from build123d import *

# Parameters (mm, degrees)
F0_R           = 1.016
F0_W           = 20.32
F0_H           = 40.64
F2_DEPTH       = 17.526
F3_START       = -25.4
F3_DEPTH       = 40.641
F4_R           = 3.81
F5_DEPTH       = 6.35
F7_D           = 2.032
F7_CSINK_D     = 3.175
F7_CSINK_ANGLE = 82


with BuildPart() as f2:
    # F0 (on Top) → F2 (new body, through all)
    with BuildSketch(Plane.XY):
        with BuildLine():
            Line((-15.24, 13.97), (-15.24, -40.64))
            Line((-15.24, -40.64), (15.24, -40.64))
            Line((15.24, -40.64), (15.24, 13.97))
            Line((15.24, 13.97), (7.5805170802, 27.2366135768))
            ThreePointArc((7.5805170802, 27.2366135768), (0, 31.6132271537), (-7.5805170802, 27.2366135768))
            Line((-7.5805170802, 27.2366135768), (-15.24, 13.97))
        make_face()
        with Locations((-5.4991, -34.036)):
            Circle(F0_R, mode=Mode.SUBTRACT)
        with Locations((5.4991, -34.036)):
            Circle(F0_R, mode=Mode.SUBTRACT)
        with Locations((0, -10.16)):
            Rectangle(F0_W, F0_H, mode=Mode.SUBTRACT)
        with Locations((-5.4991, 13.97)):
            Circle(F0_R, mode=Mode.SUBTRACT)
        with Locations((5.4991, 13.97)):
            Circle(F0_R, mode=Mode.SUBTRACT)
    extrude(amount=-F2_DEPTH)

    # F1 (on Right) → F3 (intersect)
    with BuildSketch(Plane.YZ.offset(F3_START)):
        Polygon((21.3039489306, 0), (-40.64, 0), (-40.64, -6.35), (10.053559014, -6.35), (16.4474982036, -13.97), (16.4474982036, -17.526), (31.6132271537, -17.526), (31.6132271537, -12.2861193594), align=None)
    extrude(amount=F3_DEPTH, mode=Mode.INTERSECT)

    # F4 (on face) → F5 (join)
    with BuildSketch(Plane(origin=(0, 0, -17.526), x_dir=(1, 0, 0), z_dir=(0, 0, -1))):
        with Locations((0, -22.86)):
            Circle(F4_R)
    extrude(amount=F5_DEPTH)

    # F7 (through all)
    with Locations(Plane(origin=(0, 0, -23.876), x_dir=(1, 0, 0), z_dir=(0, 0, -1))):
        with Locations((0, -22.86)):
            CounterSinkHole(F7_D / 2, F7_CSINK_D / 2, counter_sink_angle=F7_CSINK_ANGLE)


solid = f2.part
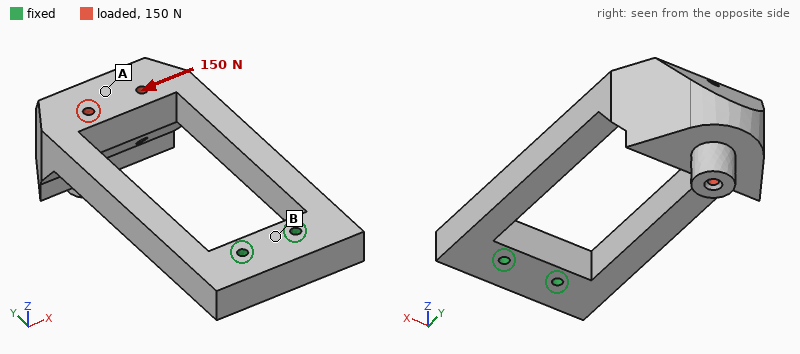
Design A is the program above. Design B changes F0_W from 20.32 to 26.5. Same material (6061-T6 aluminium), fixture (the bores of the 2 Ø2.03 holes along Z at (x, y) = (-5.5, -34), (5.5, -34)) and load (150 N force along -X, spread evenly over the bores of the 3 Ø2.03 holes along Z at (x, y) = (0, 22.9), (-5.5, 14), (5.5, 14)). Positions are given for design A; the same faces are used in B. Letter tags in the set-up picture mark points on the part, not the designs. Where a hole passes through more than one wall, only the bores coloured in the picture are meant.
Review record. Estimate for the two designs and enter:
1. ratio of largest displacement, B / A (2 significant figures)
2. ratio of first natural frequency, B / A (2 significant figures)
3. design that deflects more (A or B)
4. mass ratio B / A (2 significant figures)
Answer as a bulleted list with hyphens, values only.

- 8.3
- 0.60
- B
- 0.85
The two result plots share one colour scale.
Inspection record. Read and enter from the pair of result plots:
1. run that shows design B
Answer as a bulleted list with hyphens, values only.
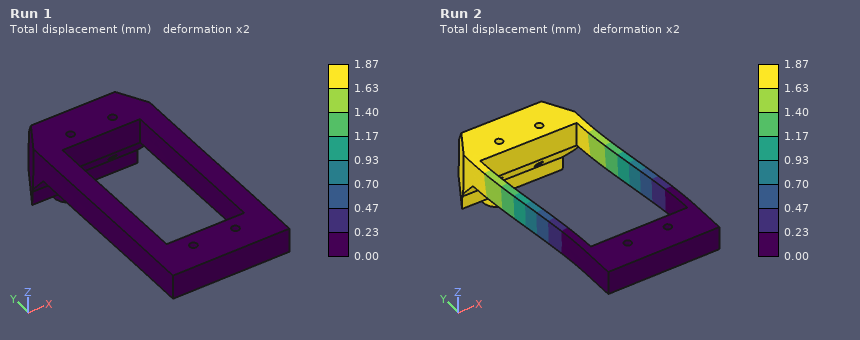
- Run 2
